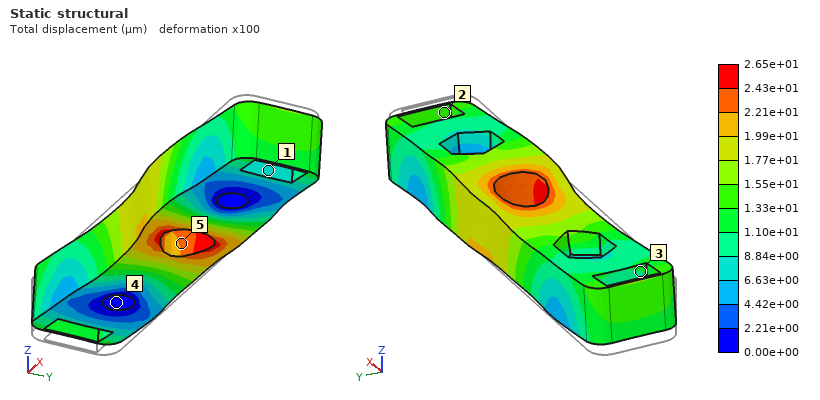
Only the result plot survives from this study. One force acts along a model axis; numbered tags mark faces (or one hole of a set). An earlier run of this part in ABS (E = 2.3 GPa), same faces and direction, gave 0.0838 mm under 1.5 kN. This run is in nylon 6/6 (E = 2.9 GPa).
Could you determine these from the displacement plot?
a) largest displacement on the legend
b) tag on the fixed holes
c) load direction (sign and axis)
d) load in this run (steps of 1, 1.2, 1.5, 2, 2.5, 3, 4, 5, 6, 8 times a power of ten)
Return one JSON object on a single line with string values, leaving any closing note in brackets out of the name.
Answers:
{"largest displacement on the legend": "2.65e+01 µm", "tag on the fixed holes": "4", "load direction": "+X", "load in this run": "600 N"}
